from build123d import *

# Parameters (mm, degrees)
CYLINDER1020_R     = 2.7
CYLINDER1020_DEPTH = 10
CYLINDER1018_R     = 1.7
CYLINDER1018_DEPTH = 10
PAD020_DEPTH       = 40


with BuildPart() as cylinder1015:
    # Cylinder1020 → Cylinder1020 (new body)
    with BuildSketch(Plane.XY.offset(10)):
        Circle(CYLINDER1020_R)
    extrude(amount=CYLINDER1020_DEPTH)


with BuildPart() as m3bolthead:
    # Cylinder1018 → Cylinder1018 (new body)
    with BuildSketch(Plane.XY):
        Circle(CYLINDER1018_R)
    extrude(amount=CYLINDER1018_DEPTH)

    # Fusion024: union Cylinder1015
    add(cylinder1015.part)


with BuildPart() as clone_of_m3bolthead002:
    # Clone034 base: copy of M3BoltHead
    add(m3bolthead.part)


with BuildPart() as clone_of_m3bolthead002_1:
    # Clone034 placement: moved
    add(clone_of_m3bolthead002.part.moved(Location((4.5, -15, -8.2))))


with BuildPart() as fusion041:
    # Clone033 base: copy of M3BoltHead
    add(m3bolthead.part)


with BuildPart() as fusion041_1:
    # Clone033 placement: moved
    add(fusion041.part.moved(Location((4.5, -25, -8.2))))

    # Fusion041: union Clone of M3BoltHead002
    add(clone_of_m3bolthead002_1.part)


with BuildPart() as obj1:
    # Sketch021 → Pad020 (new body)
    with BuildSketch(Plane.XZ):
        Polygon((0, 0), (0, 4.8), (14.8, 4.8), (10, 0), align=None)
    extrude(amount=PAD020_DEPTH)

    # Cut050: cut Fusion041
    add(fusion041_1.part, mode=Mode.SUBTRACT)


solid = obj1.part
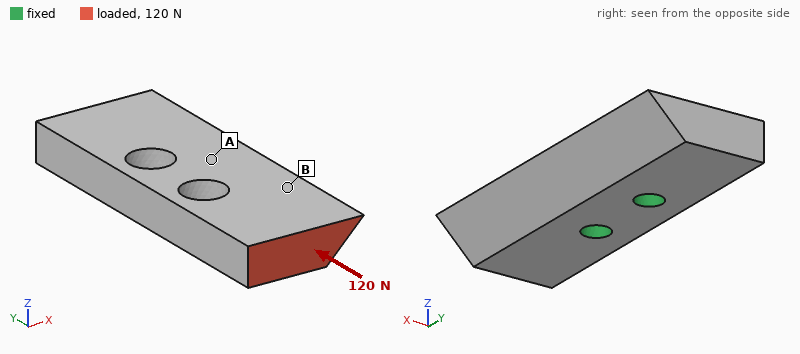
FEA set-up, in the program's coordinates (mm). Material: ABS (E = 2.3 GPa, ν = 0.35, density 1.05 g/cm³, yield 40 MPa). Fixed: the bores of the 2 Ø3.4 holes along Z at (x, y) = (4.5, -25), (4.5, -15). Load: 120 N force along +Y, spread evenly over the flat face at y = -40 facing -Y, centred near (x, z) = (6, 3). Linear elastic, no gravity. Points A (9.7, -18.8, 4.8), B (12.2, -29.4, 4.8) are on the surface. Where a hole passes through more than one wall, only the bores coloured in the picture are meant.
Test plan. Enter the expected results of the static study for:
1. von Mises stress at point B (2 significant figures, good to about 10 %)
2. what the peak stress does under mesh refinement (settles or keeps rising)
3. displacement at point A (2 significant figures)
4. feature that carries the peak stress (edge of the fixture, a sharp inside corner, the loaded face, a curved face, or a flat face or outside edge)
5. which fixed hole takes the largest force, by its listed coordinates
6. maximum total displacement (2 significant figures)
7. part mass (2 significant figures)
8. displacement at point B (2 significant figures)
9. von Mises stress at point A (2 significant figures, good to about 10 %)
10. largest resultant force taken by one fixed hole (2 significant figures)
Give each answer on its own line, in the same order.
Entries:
2.7 MPa
keeps rising
8.3 µm
edge of the fixture
(4.5, -25)
55 µm
2.3 g
25 µm
1.3 MPa
85 N
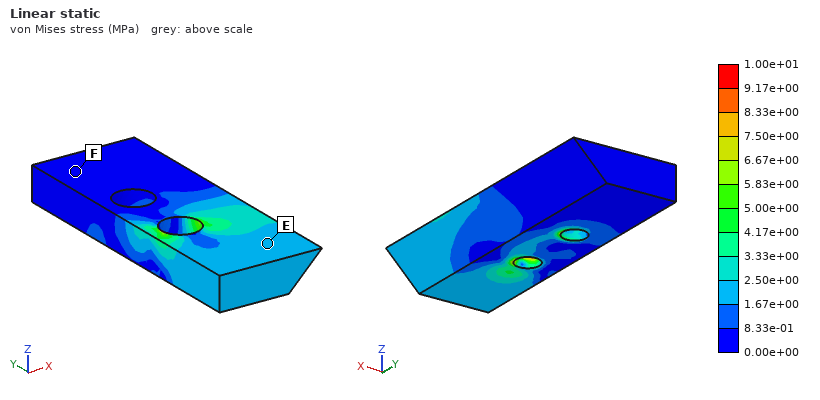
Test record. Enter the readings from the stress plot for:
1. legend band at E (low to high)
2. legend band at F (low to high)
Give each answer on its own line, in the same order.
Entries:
1.67e+00 to 2.50e+00 MPa
0.00e+00 to 8.33e-01 MPa
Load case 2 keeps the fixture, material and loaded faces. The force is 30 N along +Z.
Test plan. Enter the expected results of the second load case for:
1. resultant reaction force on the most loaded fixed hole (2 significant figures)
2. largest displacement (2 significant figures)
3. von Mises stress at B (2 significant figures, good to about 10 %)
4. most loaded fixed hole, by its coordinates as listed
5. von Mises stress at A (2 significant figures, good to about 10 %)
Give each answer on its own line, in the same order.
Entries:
72 N
0.27 mm
5.9 MPa
(4.5, -25)
2.4 MPa
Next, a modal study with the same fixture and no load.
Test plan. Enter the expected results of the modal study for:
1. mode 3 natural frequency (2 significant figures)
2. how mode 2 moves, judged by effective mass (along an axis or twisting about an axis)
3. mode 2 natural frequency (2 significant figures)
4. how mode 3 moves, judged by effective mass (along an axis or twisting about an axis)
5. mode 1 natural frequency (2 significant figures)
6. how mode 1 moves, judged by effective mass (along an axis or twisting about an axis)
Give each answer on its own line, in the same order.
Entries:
5000 Hz
along Z
3400 Hz
along X
3200 Hz
twisting about X
